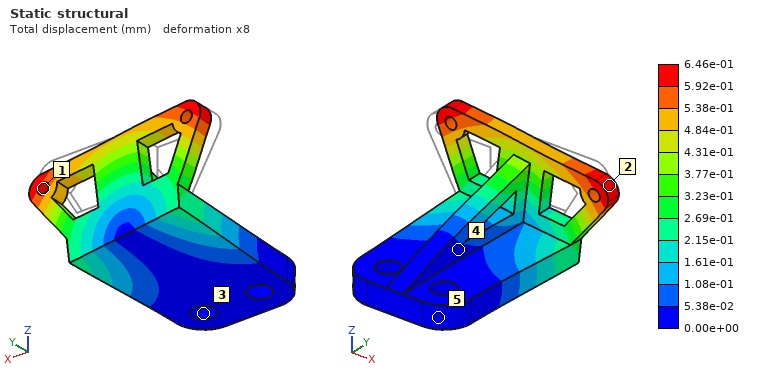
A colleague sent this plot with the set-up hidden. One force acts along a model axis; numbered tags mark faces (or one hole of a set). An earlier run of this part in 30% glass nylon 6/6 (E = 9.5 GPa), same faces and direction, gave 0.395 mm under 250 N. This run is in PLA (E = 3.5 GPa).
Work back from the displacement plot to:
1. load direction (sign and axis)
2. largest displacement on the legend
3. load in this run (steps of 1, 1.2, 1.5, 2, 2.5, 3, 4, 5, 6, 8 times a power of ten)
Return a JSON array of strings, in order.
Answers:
["+X", "6.46e-01 mm", "150 N"]
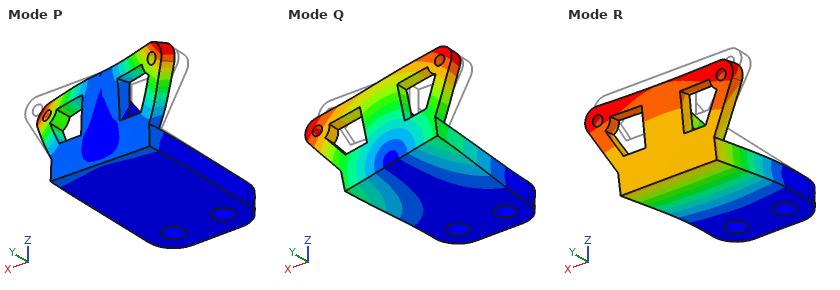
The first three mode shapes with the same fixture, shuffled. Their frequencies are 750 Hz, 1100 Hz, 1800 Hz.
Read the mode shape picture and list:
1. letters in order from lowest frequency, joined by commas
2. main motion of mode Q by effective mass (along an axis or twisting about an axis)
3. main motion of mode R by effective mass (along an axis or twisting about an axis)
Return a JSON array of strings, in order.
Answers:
["R, Q, P", "along X", "along Z"]
